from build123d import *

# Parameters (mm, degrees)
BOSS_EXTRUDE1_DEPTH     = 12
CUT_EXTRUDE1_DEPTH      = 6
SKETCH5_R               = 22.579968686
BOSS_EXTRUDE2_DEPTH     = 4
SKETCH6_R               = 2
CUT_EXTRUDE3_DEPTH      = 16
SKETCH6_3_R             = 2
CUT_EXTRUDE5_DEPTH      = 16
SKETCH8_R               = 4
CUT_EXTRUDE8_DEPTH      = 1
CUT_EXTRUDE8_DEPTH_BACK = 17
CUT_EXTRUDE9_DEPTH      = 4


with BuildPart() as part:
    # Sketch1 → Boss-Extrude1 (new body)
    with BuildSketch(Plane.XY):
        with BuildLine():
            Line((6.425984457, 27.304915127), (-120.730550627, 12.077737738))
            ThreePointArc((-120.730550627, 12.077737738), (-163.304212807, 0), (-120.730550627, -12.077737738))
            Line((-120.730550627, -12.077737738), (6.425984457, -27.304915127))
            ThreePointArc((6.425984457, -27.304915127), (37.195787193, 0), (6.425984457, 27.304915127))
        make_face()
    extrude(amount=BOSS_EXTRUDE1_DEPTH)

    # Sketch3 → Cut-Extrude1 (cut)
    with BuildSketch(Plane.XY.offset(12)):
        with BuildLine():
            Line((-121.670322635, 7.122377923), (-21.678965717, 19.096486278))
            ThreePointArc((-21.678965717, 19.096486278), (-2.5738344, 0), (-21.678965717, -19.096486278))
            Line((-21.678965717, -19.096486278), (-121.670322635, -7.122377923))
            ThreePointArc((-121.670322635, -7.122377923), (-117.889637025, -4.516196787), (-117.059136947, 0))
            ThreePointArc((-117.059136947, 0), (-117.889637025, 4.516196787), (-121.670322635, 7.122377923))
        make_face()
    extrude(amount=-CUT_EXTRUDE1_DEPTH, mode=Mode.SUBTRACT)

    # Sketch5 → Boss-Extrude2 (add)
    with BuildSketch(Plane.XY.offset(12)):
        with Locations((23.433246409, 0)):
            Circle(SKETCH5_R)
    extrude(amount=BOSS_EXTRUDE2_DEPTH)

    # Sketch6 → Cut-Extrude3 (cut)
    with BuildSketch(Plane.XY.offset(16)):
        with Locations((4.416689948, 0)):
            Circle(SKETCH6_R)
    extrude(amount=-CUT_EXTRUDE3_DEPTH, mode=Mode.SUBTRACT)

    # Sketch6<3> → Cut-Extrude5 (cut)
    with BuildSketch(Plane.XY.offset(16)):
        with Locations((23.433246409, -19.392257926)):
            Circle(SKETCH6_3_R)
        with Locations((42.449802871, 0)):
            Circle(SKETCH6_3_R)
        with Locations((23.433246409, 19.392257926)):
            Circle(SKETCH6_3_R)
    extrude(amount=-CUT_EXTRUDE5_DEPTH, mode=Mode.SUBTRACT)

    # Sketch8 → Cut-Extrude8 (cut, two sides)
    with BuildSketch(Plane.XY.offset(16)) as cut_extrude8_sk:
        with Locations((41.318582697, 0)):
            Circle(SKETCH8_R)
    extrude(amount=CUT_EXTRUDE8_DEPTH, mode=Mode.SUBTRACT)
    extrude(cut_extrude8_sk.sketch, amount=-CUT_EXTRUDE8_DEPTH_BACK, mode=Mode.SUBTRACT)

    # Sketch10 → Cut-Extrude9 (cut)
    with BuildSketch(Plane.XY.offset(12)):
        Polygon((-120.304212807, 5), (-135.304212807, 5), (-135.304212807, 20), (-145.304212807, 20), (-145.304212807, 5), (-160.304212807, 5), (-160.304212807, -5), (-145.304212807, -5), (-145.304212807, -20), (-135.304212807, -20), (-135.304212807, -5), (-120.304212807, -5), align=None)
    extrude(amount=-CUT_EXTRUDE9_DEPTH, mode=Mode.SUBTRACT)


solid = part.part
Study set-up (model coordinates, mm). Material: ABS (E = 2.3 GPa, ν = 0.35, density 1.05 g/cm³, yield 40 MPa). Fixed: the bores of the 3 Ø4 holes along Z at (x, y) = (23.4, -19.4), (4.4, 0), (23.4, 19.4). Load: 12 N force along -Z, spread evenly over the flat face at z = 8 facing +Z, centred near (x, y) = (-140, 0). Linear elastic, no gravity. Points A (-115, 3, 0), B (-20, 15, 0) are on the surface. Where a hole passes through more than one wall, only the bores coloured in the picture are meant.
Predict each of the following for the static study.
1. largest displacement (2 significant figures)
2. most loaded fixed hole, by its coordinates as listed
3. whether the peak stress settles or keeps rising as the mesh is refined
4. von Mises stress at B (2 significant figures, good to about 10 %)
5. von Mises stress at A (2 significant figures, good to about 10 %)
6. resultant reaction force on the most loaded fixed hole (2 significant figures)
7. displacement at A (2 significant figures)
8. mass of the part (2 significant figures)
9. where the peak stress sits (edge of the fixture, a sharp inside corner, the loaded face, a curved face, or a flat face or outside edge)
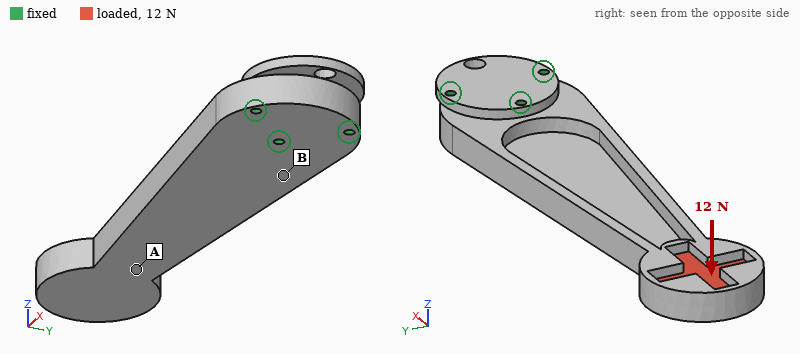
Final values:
2.2 mm
(4.4, 0)
keeps rising
1.9 MPa
0.65 MPa
67 N
1.3 mm
84 g
edge of the fixture
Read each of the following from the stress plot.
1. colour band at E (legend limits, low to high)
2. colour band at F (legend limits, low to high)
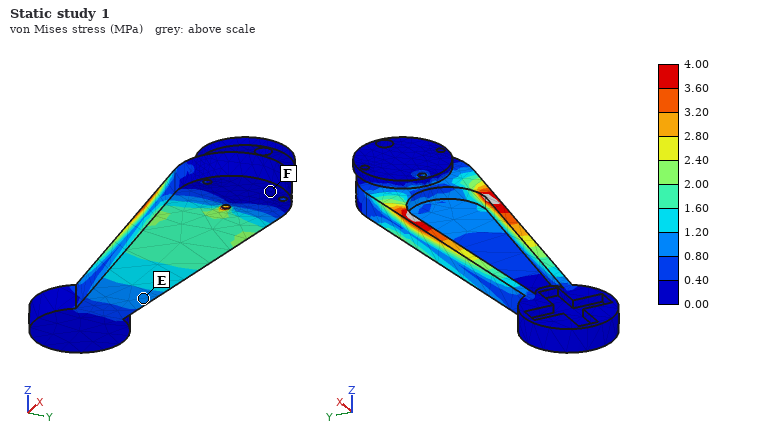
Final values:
0.80 to 1.20 MPa
0.00 to 0.40 MPa
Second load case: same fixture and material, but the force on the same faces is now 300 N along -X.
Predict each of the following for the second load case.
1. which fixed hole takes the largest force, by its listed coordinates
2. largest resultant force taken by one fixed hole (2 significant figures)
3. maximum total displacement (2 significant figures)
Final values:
(4.4, 0)
110 N
2.4 mm
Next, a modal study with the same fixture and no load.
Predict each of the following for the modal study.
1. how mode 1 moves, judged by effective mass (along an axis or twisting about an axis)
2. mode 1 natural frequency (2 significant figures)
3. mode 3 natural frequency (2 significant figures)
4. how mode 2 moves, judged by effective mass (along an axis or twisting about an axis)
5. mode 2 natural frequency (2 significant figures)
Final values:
along Z
87 Hz
450 Hz
along Y
350 Hz
